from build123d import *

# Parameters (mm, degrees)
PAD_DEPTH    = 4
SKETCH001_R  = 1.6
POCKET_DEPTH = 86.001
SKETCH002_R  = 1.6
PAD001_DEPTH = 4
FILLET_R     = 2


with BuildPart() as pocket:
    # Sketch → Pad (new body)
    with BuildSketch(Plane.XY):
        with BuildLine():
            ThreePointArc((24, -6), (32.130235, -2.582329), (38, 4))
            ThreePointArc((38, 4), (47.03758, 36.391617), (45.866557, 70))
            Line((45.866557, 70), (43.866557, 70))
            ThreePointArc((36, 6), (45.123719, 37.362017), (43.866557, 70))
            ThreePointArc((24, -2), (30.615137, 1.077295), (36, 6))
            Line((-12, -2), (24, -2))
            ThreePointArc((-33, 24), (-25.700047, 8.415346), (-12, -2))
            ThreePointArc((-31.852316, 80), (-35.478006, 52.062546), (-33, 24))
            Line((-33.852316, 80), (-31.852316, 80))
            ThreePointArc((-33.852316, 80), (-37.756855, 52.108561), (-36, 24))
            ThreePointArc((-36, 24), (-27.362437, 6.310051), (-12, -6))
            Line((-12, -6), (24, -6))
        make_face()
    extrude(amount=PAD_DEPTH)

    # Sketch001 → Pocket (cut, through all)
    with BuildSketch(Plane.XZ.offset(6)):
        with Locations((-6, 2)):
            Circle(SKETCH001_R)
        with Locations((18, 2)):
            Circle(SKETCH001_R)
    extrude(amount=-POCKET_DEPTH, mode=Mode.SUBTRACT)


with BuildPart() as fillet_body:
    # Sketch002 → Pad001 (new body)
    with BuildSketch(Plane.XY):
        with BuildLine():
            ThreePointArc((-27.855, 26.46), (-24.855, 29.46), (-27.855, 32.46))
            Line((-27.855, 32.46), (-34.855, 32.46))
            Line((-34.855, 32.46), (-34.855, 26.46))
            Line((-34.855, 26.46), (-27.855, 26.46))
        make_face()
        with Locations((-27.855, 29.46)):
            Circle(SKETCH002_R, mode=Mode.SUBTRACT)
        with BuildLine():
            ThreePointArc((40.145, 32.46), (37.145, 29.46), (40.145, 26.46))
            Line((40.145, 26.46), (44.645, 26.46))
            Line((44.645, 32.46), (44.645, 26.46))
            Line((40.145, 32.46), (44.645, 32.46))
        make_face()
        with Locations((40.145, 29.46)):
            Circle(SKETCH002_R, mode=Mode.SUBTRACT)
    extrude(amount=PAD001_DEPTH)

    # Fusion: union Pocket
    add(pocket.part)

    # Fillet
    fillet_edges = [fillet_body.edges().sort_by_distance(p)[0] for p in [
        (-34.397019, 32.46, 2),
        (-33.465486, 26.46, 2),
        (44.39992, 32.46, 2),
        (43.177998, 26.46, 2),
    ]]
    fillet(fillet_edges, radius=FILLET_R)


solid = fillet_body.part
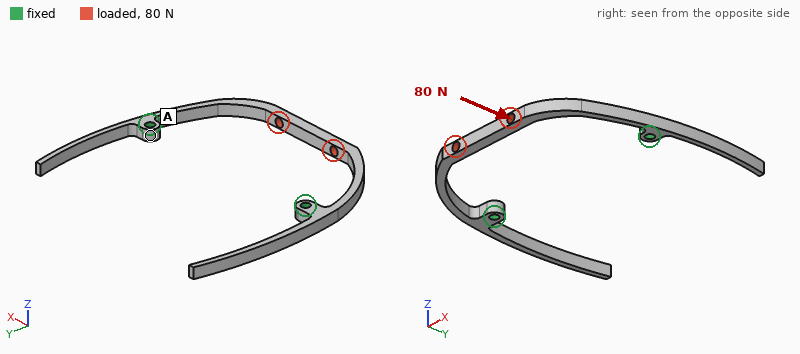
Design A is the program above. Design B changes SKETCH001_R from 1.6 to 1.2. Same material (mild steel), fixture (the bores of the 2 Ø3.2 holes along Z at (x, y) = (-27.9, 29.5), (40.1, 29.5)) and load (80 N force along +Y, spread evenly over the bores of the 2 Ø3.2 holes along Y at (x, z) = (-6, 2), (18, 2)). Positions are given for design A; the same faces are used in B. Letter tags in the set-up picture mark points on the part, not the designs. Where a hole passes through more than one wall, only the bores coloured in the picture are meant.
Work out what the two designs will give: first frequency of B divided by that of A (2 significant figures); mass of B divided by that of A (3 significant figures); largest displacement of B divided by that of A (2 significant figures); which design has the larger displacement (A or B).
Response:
1.0
1.01
0.91
A
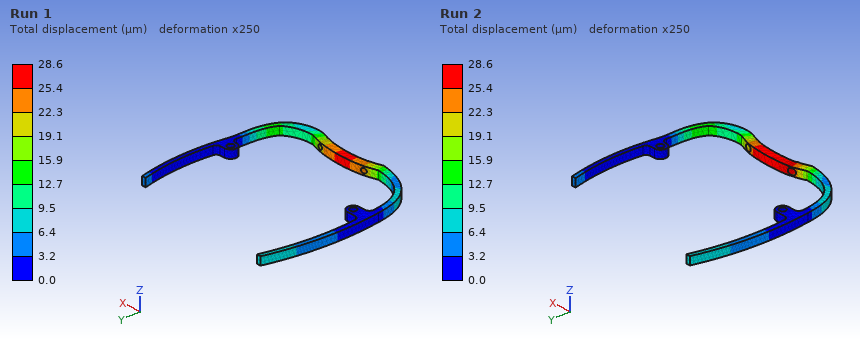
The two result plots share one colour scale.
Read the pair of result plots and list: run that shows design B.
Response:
Run 1
